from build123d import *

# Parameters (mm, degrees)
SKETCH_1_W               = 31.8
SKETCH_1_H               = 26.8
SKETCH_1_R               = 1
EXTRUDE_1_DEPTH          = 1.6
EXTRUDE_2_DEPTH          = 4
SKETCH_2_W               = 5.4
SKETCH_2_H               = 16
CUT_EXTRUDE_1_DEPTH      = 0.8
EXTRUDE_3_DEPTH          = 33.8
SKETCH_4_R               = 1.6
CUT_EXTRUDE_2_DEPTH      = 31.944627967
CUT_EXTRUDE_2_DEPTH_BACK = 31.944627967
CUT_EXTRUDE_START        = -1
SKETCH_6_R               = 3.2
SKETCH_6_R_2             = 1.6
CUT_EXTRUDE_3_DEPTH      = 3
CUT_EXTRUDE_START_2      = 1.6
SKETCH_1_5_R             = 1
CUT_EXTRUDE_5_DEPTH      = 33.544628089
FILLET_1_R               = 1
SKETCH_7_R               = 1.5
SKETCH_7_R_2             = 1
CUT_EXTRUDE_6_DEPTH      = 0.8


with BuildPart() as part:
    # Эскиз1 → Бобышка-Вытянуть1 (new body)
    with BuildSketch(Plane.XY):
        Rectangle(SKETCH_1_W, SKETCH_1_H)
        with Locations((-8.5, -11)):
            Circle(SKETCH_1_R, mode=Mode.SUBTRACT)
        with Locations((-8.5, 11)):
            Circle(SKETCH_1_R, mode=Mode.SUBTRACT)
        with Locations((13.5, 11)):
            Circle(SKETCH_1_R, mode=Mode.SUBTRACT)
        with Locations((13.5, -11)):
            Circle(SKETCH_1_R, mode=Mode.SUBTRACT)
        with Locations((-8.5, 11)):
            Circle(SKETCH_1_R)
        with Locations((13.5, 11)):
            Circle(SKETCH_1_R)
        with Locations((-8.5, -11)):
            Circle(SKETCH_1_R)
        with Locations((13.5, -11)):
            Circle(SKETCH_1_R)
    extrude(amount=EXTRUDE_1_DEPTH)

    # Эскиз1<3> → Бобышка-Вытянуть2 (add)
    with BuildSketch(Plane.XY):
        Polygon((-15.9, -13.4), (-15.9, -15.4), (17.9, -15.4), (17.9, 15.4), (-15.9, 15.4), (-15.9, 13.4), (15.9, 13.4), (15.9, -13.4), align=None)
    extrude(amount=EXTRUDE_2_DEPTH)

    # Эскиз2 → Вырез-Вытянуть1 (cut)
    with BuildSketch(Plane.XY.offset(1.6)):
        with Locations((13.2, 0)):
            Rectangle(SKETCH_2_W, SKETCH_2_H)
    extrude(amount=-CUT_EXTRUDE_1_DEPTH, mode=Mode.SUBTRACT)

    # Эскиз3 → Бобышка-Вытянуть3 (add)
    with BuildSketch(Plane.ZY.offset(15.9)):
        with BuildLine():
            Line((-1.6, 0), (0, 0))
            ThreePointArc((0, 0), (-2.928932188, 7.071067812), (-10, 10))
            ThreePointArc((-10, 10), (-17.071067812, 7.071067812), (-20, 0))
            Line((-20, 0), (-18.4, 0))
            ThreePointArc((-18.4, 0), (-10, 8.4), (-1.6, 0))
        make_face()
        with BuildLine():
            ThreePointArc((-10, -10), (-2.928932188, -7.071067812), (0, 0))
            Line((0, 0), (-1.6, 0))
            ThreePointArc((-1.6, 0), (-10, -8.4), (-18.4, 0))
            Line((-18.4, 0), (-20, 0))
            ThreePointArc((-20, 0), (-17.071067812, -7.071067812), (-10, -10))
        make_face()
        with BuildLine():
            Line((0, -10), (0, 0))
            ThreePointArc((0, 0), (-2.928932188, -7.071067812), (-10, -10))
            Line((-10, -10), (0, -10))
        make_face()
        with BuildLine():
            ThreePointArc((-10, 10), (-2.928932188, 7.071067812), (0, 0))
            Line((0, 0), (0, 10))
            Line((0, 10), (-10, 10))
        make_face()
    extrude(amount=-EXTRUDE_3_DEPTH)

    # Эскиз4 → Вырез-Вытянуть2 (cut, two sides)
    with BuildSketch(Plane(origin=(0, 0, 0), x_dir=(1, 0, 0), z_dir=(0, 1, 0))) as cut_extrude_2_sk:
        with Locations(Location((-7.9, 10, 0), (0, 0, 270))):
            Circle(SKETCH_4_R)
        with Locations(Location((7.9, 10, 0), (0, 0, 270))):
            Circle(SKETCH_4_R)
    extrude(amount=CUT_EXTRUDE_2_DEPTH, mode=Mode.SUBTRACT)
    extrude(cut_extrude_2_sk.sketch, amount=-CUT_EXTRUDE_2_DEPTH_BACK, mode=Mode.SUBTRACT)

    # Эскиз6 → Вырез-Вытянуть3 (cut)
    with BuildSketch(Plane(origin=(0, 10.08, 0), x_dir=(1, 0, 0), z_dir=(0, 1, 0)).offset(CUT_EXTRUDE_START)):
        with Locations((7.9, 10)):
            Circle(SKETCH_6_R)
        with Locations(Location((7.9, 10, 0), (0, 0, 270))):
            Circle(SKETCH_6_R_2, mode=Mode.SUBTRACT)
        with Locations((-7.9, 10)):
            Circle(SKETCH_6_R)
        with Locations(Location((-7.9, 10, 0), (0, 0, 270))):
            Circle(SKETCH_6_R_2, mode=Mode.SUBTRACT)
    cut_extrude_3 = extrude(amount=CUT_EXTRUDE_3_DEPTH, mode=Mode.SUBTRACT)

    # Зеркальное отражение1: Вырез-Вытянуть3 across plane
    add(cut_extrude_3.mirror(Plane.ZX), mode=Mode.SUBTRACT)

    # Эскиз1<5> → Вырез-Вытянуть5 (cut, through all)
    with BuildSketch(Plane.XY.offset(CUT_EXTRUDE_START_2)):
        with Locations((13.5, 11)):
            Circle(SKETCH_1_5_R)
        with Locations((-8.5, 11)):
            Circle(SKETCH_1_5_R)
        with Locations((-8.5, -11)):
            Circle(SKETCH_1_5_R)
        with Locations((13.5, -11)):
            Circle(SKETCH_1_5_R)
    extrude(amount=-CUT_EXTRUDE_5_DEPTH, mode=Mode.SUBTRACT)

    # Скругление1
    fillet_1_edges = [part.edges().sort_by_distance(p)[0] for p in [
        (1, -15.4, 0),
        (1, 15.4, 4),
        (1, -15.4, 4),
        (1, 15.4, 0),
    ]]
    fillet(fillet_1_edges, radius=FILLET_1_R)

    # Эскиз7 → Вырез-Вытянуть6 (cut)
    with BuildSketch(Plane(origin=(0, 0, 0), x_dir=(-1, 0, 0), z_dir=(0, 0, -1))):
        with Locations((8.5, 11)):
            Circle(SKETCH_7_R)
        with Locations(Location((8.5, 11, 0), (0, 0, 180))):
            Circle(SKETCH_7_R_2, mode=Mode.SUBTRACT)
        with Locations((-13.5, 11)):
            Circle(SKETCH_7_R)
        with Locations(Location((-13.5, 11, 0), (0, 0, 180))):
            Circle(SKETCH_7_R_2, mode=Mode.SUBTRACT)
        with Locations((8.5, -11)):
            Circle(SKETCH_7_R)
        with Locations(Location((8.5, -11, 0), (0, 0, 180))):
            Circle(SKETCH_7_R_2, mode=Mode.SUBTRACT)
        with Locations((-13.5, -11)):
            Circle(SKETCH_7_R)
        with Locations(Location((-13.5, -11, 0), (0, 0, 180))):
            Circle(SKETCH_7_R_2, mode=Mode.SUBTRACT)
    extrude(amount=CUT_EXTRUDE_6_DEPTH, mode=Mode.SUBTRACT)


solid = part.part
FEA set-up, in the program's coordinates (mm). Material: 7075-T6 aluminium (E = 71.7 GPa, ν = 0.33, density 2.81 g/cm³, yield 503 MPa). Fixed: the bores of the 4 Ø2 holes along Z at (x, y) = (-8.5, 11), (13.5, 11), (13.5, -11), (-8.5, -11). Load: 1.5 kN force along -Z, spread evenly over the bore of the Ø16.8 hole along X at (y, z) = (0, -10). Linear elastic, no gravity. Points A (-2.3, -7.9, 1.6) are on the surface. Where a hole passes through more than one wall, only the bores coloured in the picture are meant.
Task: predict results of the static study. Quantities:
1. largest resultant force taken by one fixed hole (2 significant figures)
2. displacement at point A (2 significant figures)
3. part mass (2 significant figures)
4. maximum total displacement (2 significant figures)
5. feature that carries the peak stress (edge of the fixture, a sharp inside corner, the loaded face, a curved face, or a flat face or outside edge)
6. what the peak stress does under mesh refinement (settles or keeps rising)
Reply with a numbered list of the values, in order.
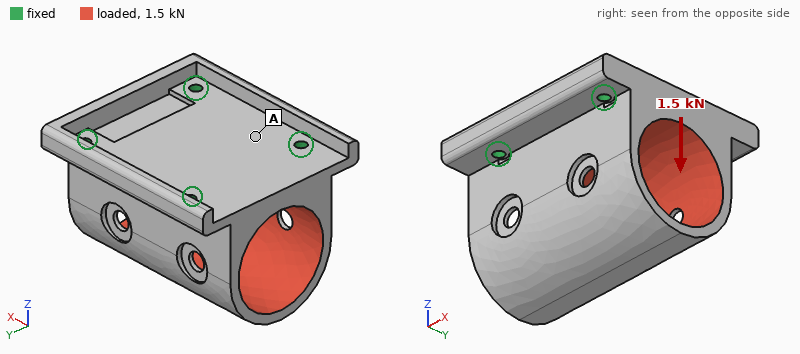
1. 460 N
2. 5.1 µm
3. 18 g
4. 12 µm
5. edge of the fixture
6. keeps rising
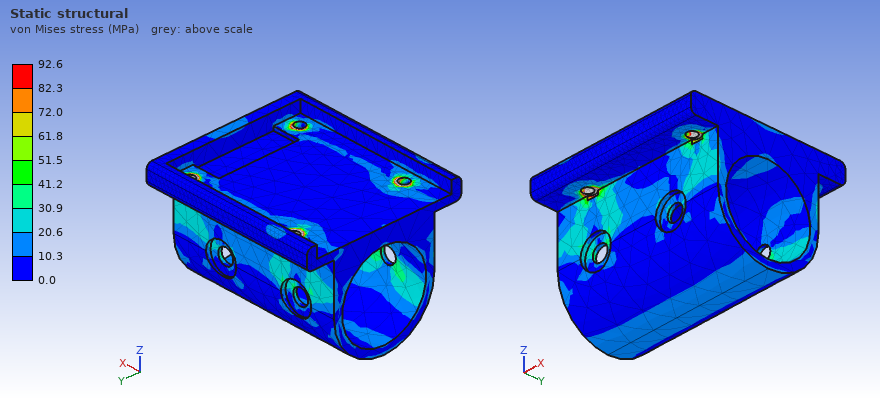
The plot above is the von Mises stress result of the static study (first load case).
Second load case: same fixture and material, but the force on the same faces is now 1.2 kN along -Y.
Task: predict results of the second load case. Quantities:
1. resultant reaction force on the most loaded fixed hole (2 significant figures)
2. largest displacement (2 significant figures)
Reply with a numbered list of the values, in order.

1. 470 N
2. 55 µm
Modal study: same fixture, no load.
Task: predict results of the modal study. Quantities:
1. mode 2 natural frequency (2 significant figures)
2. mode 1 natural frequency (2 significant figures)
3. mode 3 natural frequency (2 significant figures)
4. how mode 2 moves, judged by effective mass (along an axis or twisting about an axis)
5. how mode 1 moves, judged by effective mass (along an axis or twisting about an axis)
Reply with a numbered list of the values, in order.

1. 15 kHz
2. 8800 Hz
3. 17 kHz
4. along X
5. along Y
